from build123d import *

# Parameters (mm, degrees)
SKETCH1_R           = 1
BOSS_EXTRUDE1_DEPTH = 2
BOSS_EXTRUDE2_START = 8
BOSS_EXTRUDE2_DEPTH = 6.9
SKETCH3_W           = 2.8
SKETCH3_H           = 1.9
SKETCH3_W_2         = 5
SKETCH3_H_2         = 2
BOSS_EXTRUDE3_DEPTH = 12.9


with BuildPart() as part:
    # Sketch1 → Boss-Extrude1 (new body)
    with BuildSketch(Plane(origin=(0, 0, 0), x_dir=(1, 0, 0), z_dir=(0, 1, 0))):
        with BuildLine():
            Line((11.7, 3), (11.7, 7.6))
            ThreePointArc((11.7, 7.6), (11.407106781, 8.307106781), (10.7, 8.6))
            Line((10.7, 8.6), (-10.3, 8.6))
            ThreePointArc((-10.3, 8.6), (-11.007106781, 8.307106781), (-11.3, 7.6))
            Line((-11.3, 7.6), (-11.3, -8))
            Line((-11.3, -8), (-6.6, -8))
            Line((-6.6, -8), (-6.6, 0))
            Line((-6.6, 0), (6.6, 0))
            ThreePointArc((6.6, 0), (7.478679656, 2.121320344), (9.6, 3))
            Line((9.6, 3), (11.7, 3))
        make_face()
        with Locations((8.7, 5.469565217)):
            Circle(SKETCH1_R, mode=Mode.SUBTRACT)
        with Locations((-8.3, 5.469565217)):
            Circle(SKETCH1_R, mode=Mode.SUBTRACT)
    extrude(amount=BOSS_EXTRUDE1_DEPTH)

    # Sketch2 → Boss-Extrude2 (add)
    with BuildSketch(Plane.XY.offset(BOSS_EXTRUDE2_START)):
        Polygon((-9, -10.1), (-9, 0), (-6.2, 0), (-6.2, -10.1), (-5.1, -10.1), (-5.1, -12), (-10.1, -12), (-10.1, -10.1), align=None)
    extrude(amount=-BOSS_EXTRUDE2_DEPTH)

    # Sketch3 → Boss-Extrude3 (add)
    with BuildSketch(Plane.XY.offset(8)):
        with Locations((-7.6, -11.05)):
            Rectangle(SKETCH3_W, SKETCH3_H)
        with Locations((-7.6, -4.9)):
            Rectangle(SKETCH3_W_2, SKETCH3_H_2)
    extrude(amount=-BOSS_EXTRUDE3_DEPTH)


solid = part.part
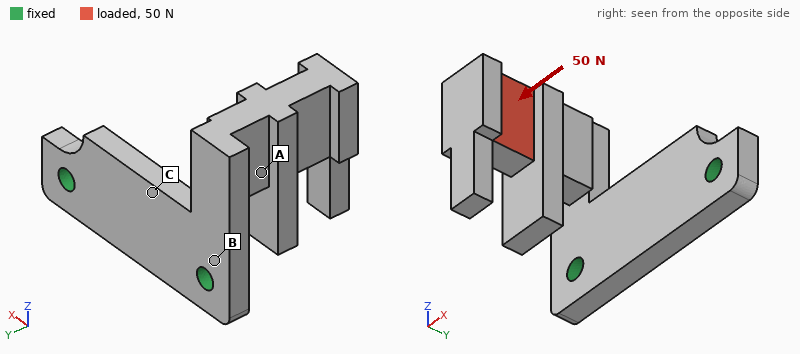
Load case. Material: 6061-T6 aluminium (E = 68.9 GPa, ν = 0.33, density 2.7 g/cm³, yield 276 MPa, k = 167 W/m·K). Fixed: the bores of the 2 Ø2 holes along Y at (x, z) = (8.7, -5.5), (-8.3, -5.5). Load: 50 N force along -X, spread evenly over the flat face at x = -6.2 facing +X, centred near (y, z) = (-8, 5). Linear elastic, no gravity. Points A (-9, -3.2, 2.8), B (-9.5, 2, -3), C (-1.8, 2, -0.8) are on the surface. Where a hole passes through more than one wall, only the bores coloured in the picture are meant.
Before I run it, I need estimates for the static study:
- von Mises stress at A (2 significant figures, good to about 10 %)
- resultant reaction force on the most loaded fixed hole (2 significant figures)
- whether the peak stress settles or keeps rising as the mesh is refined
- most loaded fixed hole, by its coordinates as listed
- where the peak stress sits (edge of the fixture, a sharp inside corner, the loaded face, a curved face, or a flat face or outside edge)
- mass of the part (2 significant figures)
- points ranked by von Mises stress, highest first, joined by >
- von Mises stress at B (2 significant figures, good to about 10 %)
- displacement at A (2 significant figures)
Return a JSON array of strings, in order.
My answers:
["30 MPa", "42 N", "keeps rising", "(8.7, -5.5)", "a sharp inside corner", "2.2 g", "B > A > C", "90 MPa", "0.050 mm"]
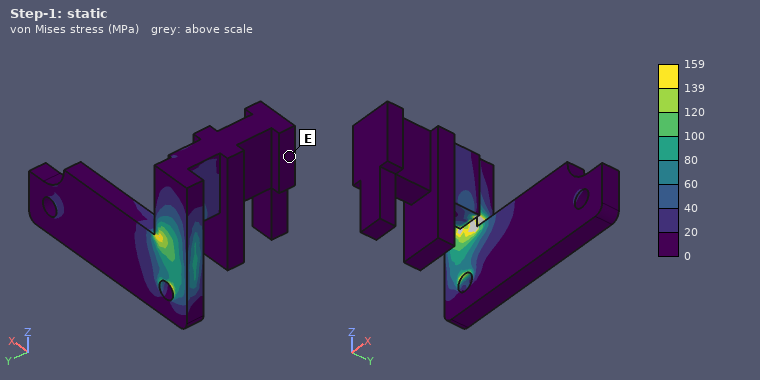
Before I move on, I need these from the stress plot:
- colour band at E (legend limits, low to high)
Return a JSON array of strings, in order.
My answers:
["0 to 20 MPa"]
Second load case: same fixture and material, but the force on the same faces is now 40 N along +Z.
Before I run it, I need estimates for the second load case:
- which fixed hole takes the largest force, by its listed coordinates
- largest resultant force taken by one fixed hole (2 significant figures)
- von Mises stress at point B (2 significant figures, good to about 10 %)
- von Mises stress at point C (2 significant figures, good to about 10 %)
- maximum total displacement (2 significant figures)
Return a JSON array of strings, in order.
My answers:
["(-8.3, -5.5)", "36 N", "75 MPa", "14 MPa", "0.16 mm"]
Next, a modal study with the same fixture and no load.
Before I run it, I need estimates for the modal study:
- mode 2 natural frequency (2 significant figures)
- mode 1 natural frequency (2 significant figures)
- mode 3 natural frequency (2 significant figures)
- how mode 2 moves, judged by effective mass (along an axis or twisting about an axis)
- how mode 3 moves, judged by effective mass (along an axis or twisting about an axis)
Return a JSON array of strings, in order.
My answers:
["3600 Hz", "2900 Hz", "12 kHz", "along X", "along Y"]
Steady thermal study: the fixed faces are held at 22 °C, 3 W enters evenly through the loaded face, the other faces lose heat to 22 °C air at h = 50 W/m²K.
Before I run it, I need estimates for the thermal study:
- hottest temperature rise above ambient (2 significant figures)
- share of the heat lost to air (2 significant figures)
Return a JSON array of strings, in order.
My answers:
["18 K", "14 %"]
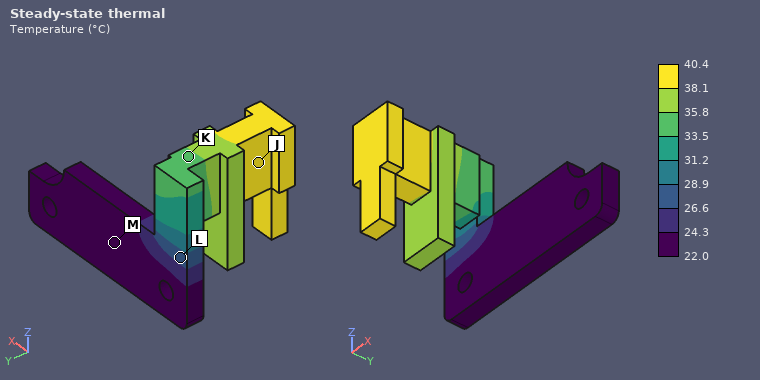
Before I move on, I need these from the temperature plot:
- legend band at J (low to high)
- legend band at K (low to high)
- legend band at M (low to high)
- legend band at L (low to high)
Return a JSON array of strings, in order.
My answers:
["38.1 to 40.4 °C", "33.5 to 35.8 °C", "22.0 to 24.3 °C", "26.6 to 28.9 °C"]
